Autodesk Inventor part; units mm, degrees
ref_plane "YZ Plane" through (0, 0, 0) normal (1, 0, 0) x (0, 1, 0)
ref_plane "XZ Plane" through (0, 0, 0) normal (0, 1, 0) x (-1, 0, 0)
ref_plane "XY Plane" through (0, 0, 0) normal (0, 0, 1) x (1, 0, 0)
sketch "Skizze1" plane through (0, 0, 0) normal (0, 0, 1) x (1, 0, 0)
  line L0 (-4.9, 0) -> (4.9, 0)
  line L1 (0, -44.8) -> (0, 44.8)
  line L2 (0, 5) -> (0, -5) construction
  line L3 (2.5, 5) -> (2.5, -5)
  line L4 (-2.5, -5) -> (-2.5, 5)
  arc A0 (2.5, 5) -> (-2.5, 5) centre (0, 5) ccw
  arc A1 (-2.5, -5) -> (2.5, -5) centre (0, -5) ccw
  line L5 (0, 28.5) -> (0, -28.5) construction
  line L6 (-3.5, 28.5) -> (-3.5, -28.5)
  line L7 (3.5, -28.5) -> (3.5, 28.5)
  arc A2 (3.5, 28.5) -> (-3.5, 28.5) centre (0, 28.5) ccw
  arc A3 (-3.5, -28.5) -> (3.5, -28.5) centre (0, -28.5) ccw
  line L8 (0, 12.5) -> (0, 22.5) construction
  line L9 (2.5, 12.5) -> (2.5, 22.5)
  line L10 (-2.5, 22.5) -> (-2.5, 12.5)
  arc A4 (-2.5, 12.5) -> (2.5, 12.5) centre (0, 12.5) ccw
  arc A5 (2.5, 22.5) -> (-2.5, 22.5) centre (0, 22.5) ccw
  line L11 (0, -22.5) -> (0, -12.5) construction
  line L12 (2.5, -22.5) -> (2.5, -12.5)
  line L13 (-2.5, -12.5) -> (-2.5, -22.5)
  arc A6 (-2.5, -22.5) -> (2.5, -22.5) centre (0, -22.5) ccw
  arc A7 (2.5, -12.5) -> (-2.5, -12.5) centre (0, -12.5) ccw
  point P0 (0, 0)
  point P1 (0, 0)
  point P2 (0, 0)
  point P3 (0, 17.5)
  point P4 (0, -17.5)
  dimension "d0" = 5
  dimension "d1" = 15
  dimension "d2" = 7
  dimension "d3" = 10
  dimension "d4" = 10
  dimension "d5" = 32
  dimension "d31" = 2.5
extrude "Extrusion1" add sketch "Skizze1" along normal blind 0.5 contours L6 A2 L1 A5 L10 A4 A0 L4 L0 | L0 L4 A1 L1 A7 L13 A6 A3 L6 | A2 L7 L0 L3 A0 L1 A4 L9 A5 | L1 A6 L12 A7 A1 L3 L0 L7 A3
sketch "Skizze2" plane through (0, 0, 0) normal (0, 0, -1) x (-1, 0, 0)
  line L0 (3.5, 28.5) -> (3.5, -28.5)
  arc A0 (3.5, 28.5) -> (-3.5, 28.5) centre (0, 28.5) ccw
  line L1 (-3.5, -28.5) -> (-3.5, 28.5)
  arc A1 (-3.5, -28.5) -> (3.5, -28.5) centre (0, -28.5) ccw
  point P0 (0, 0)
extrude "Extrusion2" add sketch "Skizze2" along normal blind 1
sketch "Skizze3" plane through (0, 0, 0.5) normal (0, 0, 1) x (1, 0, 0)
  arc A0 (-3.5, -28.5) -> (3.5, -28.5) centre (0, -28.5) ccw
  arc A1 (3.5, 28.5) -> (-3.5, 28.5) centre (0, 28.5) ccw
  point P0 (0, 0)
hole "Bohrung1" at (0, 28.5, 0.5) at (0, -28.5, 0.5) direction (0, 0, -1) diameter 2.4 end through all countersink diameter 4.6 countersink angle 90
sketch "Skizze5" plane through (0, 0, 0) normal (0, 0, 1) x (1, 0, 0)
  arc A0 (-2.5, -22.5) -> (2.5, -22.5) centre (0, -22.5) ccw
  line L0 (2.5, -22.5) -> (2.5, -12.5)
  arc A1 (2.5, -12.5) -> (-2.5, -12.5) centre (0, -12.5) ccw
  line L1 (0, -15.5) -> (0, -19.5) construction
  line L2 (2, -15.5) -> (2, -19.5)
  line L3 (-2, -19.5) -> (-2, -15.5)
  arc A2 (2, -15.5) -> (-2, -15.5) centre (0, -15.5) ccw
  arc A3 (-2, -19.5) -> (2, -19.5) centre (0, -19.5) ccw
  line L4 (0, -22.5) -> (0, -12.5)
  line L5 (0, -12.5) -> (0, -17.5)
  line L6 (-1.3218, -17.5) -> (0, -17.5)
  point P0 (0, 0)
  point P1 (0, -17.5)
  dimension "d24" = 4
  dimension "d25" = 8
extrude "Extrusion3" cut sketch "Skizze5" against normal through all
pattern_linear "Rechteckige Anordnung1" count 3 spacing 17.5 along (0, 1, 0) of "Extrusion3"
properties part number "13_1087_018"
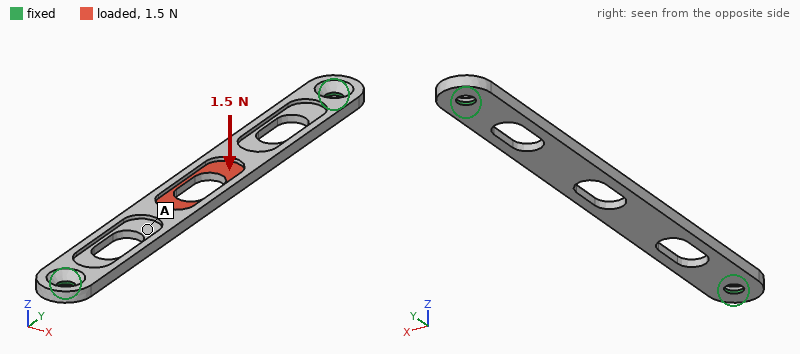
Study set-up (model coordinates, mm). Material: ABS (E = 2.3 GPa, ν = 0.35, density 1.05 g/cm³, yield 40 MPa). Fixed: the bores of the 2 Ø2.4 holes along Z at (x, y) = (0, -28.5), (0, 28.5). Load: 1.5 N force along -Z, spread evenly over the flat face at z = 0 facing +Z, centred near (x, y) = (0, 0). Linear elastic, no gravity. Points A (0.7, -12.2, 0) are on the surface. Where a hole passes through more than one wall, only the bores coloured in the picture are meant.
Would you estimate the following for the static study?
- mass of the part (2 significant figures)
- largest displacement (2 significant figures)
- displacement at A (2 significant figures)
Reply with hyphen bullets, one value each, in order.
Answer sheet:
- 0.46 g
- 0.61 mm
- 0.35 mm
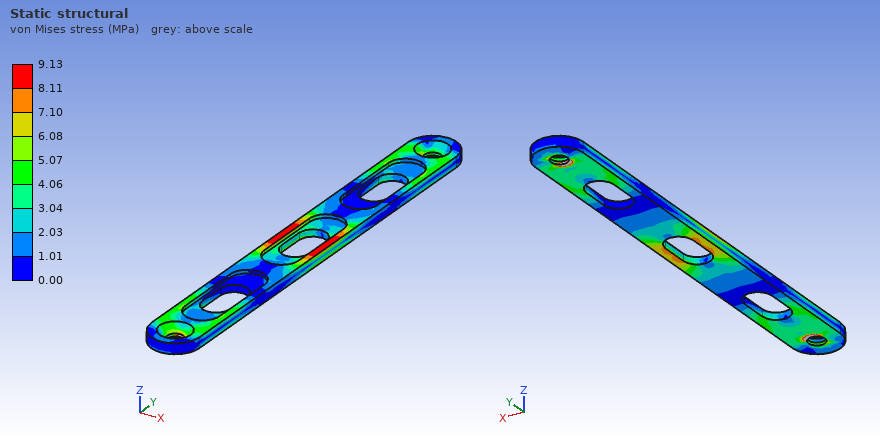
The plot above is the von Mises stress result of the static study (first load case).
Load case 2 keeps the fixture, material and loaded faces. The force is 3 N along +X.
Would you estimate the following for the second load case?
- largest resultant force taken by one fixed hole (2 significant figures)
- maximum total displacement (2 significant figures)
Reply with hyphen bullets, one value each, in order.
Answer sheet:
- 1.5 N
- 0.11 mm
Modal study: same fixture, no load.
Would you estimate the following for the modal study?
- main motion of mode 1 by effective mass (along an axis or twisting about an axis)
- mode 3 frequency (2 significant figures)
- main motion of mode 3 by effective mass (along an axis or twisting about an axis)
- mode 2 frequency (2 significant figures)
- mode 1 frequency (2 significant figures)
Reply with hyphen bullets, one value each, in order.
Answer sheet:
- along Z
- 1900 Hz
- along X
- 1700 Hz
- 620 Hz
